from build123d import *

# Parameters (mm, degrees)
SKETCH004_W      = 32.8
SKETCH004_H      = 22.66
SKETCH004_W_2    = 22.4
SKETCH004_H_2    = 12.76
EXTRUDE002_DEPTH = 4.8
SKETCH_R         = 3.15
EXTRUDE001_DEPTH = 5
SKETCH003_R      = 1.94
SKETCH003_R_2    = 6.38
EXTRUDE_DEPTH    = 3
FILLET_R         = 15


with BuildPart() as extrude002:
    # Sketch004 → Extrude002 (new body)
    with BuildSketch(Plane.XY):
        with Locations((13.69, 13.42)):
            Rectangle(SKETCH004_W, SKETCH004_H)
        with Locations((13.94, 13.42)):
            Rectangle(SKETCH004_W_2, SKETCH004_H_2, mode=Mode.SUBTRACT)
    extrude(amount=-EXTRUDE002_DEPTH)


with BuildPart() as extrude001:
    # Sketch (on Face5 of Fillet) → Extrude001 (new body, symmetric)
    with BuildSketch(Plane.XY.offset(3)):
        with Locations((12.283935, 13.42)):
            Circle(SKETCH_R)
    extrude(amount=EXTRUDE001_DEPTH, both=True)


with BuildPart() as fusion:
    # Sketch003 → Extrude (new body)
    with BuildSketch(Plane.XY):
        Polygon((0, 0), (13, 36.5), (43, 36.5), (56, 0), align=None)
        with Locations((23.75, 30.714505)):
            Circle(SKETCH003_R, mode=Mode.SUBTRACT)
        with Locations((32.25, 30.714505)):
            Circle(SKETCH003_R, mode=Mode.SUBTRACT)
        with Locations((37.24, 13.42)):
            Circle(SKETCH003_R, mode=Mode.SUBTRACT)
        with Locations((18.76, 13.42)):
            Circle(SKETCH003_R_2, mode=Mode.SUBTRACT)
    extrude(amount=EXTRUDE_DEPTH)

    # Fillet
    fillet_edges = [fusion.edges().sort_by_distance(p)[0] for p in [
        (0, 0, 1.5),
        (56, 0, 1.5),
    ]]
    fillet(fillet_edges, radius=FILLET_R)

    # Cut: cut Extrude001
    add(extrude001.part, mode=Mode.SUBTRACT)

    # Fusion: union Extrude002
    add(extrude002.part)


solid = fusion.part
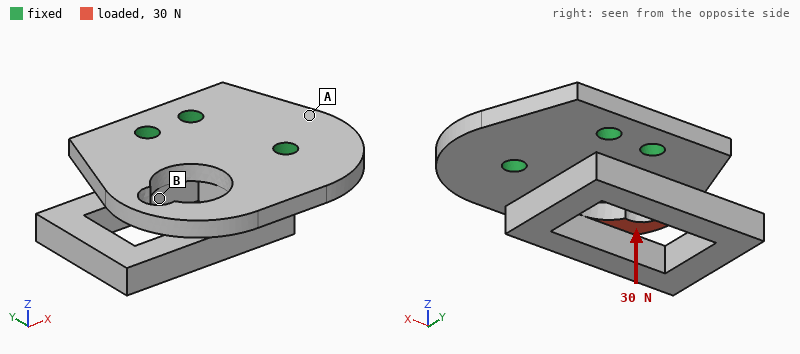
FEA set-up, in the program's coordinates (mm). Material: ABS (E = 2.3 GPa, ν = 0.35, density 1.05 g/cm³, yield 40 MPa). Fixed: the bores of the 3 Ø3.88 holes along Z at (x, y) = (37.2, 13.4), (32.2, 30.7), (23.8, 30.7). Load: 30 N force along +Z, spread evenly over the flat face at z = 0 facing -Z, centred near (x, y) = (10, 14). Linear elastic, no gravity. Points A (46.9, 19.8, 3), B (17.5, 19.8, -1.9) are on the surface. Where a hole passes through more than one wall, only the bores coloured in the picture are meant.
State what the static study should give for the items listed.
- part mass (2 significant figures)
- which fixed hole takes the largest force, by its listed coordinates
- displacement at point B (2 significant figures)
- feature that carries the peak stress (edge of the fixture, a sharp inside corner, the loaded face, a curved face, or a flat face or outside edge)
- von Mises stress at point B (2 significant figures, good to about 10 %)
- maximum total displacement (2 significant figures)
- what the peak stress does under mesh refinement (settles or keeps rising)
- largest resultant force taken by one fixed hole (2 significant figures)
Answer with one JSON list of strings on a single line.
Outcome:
["6.0 g", "(23.8, 30.7)", "0.15 mm", "edge of the fixture", "3.5 MPa", "0.63 mm", "keeps rising", "43 N"]
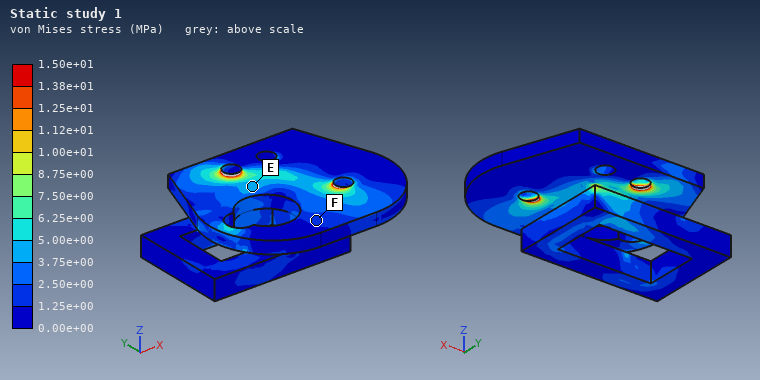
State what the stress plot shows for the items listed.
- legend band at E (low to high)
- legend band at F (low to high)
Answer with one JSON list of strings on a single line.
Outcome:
["3.75e+00 to 5.00e+00 MPa", "1.25e+00 to 2.50e+00 MPa"]
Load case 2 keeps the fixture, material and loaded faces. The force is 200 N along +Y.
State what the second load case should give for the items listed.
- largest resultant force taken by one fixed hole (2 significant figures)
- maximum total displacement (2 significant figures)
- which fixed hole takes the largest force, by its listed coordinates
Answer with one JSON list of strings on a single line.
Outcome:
["210 N", "0.32 mm", "(23.8, 30.7)"]
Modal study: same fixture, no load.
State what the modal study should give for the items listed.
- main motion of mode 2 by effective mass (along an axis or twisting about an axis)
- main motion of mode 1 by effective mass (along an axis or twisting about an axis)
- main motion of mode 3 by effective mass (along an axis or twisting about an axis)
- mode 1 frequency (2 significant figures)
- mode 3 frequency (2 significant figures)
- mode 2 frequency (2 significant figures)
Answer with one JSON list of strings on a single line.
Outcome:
["twisting about X", "along Z", "along Y", "880 Hz", "3200 Hz", "2600 Hz"]
